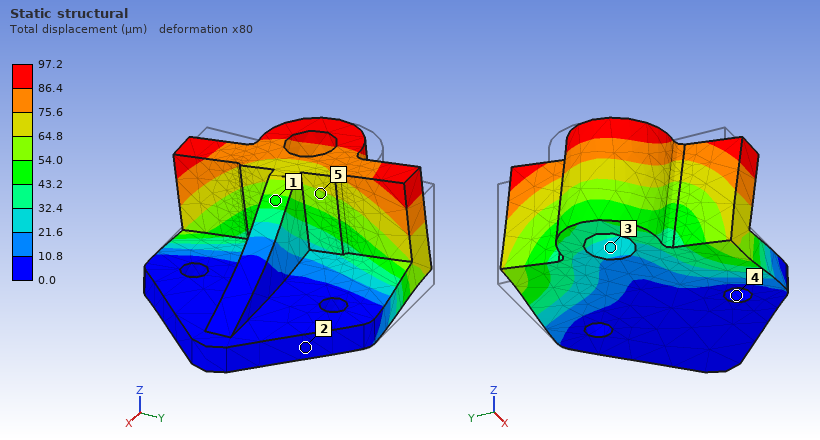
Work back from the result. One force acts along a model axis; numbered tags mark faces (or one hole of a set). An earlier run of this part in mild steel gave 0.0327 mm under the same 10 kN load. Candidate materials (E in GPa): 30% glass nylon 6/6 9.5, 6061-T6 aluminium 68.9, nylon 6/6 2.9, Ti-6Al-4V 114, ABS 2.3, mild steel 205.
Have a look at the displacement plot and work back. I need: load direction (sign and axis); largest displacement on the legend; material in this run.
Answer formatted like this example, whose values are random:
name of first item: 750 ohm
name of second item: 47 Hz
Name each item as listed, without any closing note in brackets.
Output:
load direction: -Y
largest displacement on the legend: 97.2 µm
material in this run: 6061-T6 aluminium
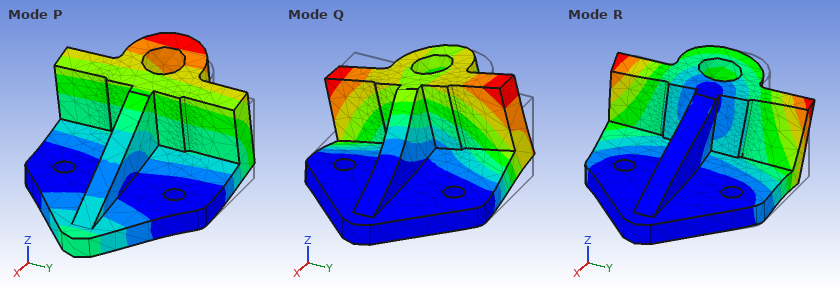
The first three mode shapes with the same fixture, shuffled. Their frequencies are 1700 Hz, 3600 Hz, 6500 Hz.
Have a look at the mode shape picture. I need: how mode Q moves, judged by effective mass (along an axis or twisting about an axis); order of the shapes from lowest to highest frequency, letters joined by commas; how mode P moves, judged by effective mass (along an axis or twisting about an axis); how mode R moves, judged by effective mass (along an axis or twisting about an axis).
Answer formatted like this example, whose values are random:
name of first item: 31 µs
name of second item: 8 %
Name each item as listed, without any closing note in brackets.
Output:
how mode Q moves, judged by effective mass: along Y
order of the shapes from lowest to highest frequency, letters joined by commas: P, Q, R
how mode P moves, judged by effective mass: along Z
how mode R moves, judged by effective mass: along Y
